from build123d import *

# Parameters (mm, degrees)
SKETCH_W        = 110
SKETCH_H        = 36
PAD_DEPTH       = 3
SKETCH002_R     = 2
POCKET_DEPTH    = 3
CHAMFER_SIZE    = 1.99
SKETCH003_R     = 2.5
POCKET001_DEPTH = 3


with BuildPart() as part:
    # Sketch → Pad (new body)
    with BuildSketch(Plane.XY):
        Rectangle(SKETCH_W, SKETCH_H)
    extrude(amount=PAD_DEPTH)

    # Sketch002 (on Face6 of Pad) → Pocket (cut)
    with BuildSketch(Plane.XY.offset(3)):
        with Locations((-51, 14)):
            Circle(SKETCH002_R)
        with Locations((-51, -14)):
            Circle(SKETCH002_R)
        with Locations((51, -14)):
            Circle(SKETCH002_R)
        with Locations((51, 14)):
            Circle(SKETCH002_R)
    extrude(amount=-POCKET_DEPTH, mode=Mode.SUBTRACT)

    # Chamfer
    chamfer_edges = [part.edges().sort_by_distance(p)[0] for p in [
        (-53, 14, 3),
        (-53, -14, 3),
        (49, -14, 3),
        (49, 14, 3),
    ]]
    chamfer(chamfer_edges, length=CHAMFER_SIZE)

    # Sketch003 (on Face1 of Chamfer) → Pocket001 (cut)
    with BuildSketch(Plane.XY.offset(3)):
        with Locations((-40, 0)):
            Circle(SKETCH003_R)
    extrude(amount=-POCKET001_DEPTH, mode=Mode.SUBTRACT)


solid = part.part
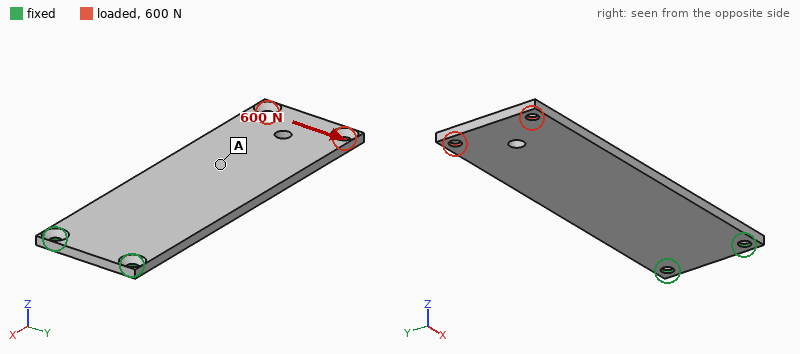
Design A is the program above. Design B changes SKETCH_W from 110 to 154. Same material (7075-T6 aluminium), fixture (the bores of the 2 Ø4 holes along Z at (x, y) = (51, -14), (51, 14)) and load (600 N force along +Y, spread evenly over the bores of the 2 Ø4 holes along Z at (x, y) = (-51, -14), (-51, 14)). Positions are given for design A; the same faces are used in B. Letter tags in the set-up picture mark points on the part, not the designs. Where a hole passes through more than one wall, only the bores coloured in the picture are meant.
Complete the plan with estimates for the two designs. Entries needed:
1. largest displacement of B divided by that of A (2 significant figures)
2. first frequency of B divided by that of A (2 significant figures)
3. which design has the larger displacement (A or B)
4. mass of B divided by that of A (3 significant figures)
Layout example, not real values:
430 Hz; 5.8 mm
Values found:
1.2; 0.71; B; 1.41
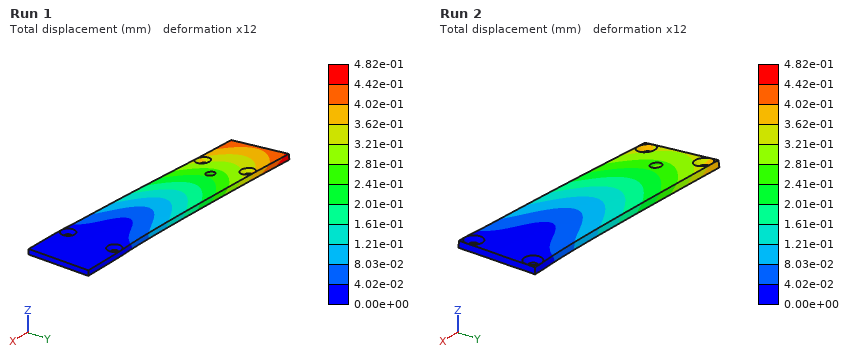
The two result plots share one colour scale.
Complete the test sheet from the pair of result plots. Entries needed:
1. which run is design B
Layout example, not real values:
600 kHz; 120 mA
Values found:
Run 1
